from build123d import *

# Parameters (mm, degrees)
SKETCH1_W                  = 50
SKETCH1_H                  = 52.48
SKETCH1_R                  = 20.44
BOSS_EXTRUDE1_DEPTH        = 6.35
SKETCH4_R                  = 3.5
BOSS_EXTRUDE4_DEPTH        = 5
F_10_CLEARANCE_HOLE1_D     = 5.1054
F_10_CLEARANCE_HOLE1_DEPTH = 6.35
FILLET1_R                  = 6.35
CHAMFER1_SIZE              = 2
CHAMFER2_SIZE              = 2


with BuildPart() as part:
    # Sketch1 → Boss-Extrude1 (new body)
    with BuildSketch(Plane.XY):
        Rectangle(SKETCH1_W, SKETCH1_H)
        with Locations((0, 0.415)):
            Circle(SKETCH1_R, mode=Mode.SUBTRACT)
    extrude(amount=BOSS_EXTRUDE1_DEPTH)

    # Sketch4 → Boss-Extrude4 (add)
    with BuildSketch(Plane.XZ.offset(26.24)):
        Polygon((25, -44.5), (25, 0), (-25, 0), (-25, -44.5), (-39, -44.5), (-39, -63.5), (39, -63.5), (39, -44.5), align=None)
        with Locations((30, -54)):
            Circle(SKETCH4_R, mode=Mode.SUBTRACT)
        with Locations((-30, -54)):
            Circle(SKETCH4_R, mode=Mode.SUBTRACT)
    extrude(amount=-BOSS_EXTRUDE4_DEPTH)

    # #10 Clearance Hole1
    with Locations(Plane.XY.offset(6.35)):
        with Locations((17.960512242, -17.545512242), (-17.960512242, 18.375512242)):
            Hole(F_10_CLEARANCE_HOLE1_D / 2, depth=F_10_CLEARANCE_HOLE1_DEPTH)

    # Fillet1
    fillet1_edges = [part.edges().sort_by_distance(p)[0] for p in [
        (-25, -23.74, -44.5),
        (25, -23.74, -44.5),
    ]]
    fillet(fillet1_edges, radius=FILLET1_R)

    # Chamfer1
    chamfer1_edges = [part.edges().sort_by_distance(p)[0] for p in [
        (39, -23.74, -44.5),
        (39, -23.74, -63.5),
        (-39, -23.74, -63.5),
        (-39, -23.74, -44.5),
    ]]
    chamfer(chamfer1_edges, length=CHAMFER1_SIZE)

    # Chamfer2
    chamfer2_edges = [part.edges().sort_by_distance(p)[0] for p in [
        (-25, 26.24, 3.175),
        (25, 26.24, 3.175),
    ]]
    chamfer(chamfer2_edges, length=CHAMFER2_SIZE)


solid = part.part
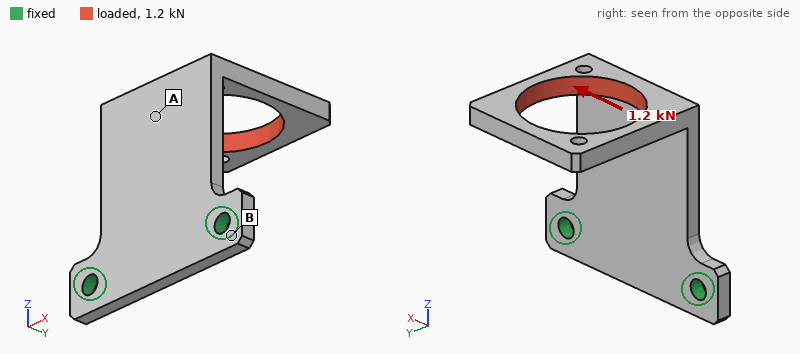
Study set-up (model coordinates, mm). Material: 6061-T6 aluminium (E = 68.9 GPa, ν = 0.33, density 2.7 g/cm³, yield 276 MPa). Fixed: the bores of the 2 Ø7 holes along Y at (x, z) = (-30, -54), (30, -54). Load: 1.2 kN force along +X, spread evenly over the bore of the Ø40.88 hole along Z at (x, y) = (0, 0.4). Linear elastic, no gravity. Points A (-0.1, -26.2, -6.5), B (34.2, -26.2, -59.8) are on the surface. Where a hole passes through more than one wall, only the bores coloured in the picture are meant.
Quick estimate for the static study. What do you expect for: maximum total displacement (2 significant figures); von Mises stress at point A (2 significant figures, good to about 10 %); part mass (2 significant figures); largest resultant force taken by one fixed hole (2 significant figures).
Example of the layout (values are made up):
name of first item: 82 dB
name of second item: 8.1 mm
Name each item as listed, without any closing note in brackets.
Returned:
maximum total displacement: 1.3 mm
von Mises stress at point A: 69 MPa
part mass: 71 g
largest resultant force taken by one fixed hole: 1.5 kN
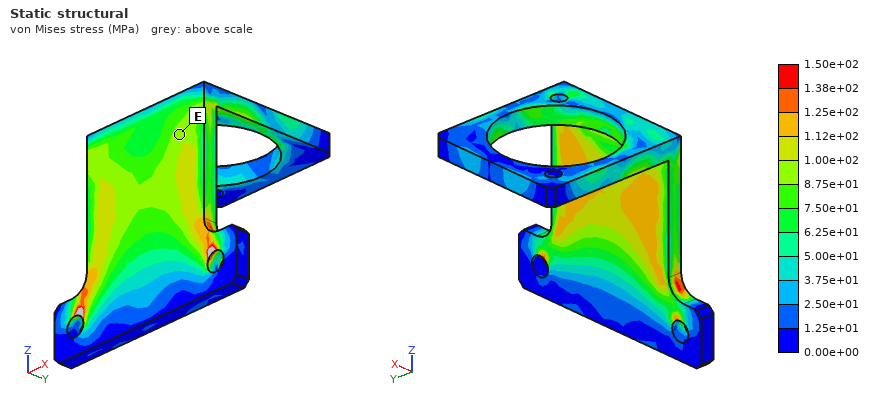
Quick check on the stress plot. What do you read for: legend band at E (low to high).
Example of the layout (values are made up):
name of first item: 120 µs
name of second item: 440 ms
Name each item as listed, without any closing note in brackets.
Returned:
legend band at E: 8.75e+01 to 1.00e+02 MPa
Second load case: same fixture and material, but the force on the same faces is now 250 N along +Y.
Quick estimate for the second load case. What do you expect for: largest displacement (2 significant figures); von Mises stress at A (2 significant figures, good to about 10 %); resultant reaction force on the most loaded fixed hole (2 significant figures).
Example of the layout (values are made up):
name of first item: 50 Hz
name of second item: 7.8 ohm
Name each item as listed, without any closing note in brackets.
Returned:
largest displacement: 0.84 mm
von Mises stress at A: 12 MPa
resultant reaction force on the most loaded fixed hole: 130 N
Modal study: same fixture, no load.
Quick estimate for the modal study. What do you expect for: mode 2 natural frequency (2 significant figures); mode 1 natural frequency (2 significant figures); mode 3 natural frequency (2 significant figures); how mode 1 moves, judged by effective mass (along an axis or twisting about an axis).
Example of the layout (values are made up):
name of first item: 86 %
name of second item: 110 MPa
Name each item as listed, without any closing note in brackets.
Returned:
mode 2 natural frequency: 1100 Hz
mode 1 natural frequency: 530 Hz
mode 3 natural frequency: 1300 Hz
how mode 1 moves, judged by effective mass: along Y
